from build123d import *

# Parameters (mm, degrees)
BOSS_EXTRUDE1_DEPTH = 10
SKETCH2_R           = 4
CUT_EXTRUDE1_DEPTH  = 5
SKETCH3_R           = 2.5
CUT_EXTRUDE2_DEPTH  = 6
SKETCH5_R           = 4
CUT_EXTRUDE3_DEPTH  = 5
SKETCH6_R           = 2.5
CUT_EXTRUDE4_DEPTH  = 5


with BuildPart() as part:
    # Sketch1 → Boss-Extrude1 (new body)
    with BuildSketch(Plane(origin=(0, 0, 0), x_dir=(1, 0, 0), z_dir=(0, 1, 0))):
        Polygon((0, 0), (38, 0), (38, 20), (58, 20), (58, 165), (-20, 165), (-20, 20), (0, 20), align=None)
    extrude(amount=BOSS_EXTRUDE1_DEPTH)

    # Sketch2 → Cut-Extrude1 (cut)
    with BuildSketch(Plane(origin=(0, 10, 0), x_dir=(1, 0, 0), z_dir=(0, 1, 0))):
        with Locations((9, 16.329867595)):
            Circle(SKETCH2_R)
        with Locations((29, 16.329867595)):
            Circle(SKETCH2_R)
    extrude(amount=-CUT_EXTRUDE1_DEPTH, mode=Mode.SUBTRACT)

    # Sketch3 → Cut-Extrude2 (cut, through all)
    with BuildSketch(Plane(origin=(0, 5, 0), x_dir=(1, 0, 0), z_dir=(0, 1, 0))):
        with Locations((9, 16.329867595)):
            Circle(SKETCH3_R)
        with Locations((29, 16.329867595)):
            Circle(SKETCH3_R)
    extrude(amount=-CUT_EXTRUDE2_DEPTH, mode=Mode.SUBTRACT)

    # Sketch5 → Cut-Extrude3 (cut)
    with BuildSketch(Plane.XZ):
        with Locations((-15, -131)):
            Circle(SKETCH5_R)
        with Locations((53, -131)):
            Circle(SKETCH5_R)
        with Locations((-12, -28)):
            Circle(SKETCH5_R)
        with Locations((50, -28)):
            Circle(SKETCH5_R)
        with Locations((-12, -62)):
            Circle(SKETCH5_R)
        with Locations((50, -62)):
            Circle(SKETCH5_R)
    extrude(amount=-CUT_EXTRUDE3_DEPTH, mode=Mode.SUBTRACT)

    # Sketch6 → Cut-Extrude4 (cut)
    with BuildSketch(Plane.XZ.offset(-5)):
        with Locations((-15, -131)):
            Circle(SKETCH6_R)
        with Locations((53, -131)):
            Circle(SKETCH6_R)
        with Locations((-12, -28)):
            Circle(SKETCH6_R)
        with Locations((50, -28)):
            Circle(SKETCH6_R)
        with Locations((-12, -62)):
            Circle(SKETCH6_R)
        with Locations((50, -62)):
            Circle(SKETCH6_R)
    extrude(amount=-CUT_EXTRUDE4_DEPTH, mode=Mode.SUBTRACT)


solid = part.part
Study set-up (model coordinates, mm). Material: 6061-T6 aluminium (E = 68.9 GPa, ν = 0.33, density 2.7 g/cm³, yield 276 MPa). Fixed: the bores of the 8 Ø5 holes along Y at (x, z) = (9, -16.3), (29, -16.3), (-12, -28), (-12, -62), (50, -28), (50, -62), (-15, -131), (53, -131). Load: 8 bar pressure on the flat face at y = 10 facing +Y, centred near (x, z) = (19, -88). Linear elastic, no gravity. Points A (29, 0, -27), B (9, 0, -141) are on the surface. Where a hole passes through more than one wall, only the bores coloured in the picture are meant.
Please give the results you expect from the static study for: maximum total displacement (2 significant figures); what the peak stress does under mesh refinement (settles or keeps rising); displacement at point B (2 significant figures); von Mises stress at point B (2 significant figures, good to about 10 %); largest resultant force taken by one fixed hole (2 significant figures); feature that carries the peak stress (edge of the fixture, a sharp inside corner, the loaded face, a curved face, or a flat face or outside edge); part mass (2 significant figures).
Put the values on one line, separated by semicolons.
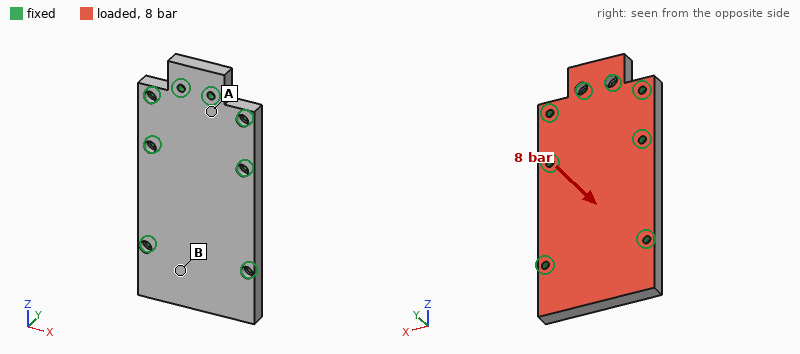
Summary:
74 µm; keeps rising; 38 µm; 25 MPa; 2.6 kN; edge of the fixture; 320 g
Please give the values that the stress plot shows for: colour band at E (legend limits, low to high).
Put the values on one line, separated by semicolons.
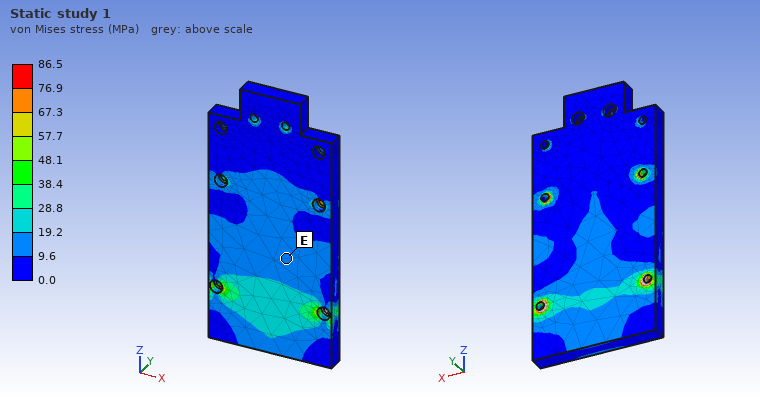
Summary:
9.6 to 19.2 MPa
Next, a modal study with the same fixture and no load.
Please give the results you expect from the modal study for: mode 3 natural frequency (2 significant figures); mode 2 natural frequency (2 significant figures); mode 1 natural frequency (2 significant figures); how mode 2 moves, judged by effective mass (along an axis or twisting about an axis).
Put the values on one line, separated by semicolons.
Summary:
7400 Hz; 5900 Hz; 3800 Hz; along Y
